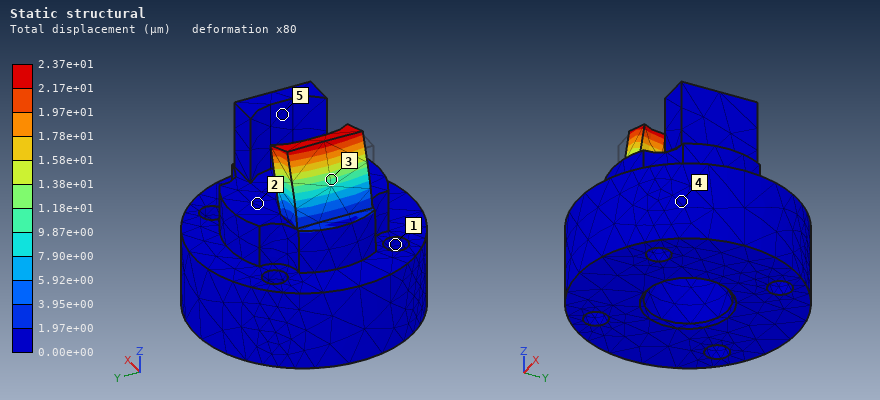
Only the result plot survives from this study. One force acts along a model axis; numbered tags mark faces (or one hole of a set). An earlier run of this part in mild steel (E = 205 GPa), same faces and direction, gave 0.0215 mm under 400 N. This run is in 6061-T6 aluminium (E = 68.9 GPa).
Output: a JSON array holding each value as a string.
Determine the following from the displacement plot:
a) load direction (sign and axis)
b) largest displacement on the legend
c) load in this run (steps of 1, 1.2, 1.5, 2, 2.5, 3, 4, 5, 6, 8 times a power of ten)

["+X", "2.37e+01 µm", "150 N"]
